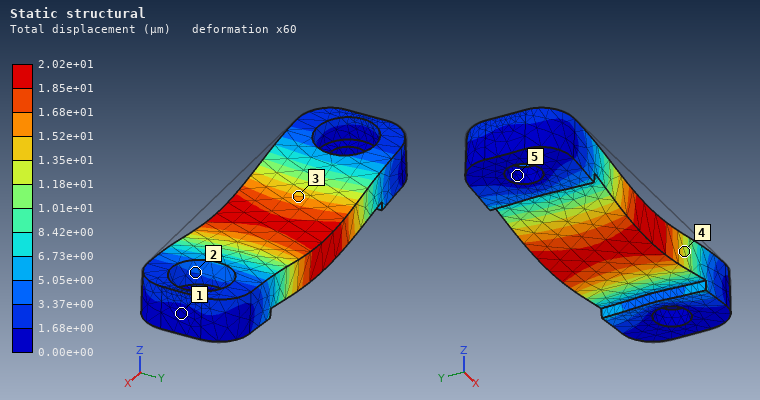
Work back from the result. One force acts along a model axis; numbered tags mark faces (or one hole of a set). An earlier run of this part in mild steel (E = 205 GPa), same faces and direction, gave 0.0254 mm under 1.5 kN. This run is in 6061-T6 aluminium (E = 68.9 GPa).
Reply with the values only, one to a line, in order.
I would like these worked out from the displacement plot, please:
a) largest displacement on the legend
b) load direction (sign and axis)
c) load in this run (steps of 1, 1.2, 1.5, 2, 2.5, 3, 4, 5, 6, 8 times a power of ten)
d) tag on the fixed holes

2.02e+01 µm
-Z
400 N
5
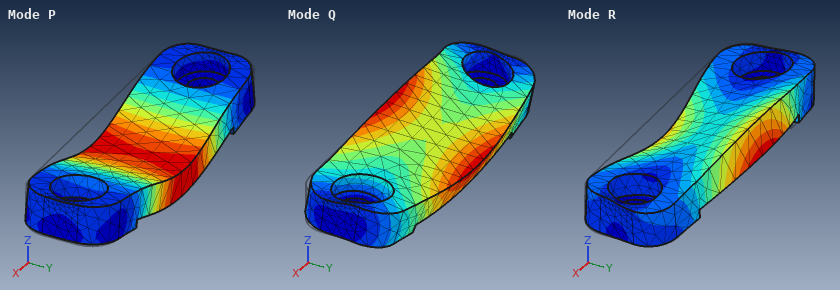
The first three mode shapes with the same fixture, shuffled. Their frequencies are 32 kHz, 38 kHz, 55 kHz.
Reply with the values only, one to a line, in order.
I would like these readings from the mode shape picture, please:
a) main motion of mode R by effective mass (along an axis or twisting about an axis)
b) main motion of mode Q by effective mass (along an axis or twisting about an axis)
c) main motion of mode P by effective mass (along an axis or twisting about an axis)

along Y
along Y
along Z
